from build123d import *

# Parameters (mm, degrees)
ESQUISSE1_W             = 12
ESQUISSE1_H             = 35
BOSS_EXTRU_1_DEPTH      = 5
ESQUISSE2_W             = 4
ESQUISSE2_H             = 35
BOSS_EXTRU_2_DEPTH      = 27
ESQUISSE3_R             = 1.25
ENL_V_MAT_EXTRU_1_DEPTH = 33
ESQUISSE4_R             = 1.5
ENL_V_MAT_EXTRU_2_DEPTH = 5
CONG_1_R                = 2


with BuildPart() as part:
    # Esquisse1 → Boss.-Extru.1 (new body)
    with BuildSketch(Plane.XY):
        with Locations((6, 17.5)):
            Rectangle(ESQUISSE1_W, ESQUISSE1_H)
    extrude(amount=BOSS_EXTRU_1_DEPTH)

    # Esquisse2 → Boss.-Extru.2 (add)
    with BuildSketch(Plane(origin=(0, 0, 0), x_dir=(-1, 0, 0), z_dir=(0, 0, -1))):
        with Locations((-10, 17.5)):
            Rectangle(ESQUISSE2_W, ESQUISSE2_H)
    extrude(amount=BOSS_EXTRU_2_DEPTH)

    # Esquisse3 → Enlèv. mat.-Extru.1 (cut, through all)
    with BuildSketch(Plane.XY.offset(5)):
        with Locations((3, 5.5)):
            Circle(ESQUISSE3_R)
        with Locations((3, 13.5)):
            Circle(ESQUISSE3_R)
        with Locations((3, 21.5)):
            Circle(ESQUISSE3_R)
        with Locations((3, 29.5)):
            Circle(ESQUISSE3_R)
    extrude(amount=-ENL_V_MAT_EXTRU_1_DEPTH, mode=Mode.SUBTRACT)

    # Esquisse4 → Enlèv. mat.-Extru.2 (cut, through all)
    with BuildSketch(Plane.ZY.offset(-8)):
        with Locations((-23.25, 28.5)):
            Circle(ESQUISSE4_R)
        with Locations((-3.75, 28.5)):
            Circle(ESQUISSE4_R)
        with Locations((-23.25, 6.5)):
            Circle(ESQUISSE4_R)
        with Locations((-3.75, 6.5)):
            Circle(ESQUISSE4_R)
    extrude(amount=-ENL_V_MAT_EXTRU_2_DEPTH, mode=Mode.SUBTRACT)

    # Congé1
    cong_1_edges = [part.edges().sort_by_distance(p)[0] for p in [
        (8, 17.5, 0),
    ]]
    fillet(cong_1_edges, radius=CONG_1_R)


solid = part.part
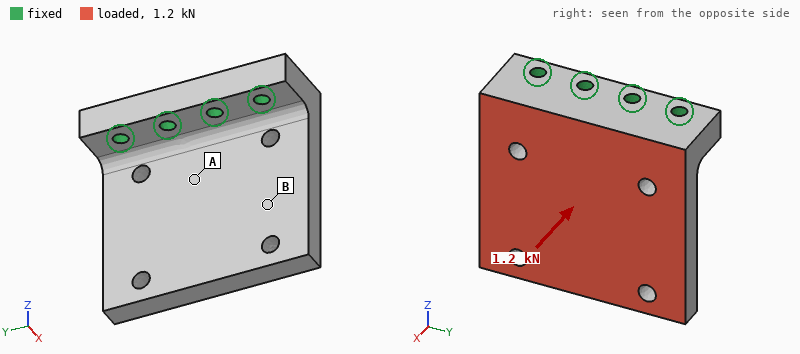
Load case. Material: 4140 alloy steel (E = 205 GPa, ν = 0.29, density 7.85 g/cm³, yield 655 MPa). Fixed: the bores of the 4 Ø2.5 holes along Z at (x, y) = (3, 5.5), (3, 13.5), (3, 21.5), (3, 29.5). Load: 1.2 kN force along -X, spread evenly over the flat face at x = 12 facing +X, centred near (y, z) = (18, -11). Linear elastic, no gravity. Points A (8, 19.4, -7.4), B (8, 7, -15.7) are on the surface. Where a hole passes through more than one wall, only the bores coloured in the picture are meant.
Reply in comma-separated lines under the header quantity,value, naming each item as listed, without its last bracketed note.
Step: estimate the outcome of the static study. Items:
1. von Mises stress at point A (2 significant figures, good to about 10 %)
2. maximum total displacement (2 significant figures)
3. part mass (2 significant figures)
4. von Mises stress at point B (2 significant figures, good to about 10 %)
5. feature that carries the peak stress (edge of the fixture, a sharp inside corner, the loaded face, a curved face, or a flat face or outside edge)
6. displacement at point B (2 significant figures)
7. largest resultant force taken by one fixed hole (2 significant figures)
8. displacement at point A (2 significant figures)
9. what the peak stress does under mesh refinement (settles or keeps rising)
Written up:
quantity,value
von Mises stress at point A,75 MPa
maximum total displacement,0.11 mm
part mass,45 g
von Mises stress at point B,24 MPa
feature that carries the peak stress,edge of the fixture
displacement at point B,0.057 mm
largest resultant force taken by one fixed hole,350 N
displacement at point A,0.023 mm
what the peak stress does under mesh refinement,keeps rising
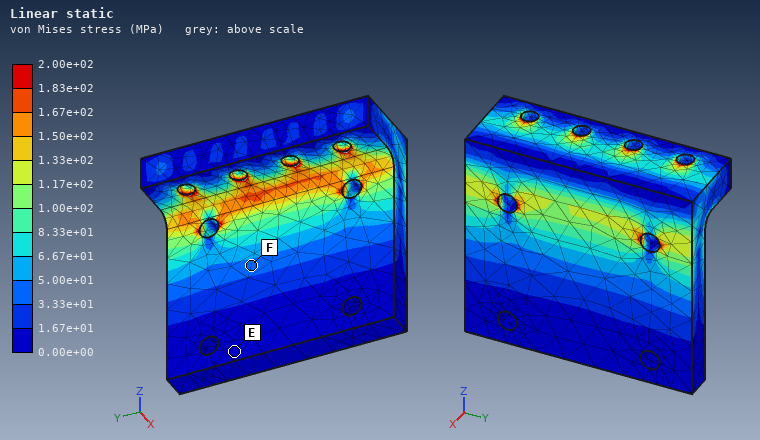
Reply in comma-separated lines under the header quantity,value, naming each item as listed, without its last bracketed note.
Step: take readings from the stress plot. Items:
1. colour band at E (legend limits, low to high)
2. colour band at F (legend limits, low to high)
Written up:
quantity,value
colour band at E,0.00e+00 to 1.67e+01 MPa
colour band at F,3.33e+01 to 5.00e+01 MPa
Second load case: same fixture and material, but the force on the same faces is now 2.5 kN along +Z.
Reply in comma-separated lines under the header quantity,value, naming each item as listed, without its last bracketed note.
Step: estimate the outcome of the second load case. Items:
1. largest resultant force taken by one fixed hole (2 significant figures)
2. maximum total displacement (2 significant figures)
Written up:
quantity,value
largest resultant force taken by one fixed hole,650 N
maximum total displacement,69 µm
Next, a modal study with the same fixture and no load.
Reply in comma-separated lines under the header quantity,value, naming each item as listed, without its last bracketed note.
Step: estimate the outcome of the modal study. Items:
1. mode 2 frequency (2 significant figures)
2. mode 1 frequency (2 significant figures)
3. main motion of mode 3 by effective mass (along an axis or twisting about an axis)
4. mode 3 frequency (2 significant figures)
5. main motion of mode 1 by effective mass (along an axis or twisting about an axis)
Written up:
quantity,value
mode 2 frequency,7500 Hz
mode 1 frequency,3500 Hz
main motion of mode 3 by effective mass,along Y
mode 3 frequency,11 kHz
main motion of mode 1 by effective mass,along X
